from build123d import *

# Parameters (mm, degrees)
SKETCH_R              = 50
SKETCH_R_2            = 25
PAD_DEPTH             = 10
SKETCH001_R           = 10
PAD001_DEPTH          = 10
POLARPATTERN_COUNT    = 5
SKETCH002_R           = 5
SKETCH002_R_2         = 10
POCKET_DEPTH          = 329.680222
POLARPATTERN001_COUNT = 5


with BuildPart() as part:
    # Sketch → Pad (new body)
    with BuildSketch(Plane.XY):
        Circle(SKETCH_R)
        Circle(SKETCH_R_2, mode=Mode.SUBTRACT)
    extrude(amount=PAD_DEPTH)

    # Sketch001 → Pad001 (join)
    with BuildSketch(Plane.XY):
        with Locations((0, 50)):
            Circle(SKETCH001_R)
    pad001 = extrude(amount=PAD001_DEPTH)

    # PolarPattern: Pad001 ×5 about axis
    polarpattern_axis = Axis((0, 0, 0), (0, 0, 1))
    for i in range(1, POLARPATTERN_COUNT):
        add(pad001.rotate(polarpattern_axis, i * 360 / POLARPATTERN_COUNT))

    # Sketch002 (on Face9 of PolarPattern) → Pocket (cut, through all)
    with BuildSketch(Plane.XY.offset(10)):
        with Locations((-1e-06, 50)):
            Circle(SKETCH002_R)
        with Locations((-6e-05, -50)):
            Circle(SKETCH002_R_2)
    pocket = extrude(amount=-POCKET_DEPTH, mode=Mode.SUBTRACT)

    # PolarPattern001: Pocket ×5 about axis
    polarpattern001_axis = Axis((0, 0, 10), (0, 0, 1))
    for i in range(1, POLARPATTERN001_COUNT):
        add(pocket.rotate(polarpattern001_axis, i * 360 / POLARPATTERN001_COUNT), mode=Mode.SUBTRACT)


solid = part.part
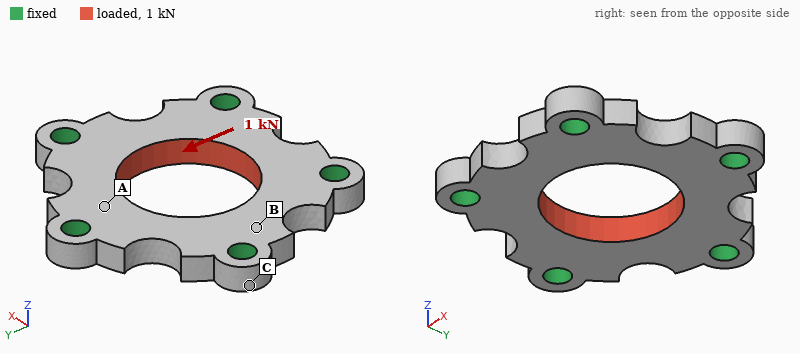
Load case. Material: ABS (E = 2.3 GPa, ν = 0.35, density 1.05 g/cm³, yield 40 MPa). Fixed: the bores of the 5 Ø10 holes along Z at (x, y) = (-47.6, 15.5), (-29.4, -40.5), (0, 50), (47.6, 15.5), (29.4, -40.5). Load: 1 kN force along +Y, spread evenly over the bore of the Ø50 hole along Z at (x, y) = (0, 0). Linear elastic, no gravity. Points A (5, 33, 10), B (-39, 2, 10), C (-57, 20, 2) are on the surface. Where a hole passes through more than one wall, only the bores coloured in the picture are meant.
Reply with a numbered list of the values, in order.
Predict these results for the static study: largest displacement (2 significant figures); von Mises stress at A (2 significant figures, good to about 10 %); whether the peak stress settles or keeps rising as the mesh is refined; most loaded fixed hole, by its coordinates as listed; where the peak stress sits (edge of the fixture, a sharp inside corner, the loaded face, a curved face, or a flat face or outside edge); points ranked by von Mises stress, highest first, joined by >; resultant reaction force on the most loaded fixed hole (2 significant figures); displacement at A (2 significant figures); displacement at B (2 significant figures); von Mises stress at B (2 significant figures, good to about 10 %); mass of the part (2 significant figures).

1. 19 µm
2. 1.2 MPa
3. keeps rising
4. (0, 50)
5. edge of the fixture
6. A > B > C
7. 310 N
8. 7.5 µm
9. 6.0 µm
10. 0.58 MPa
11. 58 g
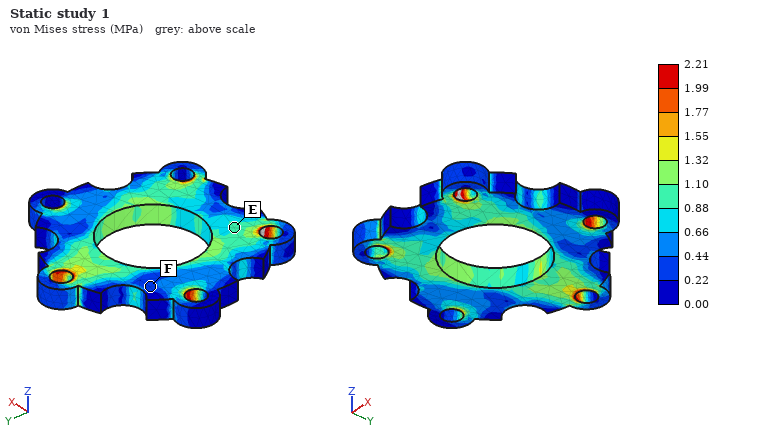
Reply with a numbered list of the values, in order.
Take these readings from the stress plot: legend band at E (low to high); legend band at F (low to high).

1. 0.88 to 1.10 MPa
2. 0.22 to 0.44 MPa
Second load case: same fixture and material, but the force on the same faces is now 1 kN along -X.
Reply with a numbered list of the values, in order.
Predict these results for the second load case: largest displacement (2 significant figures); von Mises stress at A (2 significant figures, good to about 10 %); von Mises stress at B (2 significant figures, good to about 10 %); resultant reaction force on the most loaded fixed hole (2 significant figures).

1. 19 µm
2. 0.38 MPa
3. 0.97 MPa
4. 290 N
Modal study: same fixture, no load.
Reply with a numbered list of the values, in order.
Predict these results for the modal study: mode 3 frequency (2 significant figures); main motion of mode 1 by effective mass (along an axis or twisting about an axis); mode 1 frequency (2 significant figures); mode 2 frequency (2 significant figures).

1. 4100 Hz
2. along Z
3. 3400 Hz
4. 4100 Hz
